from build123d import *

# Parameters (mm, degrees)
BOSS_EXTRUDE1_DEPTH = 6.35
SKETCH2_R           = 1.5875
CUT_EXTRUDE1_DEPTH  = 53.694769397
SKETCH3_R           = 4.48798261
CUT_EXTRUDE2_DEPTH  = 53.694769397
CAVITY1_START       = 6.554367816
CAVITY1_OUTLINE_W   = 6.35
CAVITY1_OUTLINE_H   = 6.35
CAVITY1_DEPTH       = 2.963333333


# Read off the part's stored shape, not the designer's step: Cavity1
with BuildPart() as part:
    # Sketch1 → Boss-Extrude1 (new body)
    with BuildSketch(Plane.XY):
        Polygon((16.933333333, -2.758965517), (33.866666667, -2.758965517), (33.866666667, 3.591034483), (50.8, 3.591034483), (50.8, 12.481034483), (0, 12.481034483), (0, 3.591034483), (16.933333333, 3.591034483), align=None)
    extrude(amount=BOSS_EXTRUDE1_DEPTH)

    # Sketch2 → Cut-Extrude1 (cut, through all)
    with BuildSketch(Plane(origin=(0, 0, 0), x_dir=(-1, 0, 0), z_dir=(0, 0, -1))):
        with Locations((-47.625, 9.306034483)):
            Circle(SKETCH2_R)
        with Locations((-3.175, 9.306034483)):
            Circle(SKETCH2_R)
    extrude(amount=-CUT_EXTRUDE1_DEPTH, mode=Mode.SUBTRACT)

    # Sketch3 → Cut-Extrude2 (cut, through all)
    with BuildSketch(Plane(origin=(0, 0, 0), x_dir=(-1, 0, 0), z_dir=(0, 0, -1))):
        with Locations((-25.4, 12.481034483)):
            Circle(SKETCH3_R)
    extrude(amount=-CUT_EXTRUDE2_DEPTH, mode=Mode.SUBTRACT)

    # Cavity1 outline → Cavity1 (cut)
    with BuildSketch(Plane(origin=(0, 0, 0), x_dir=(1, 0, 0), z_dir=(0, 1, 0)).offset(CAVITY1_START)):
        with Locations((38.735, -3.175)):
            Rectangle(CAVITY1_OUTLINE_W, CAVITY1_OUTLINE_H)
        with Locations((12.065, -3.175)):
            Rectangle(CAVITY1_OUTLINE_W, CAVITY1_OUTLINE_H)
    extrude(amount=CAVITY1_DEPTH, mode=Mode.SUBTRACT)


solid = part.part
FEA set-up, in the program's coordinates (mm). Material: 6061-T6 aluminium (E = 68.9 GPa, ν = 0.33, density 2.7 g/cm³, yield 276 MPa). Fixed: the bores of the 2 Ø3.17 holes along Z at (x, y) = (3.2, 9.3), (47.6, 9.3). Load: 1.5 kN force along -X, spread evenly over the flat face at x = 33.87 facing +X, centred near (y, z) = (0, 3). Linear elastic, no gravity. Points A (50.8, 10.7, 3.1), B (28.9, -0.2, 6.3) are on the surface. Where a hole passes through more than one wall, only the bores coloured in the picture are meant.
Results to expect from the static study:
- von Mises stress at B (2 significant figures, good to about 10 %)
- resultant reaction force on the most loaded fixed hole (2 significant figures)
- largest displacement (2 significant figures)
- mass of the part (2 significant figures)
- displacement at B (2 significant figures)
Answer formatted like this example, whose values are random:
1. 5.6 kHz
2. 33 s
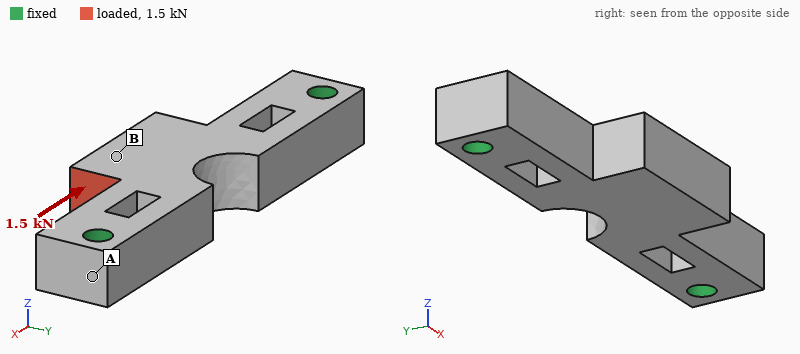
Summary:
1. 28 MPa
2. 810 N
3. 24 µm
4. 8.1 g
5. 15 µm
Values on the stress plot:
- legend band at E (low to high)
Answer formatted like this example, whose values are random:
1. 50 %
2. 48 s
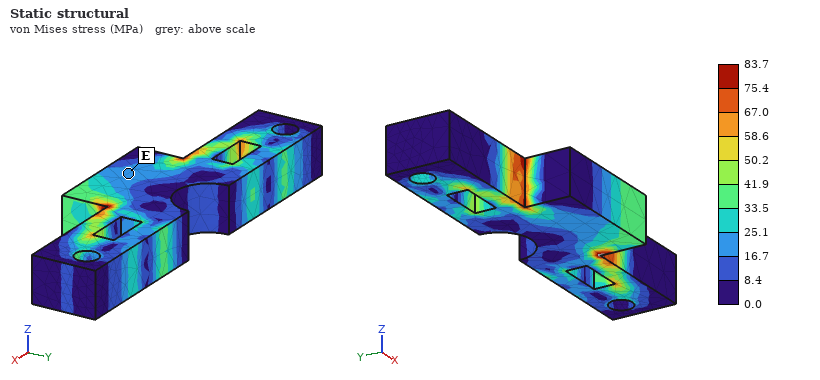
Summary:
1. 16.7 to 25.1 MPa
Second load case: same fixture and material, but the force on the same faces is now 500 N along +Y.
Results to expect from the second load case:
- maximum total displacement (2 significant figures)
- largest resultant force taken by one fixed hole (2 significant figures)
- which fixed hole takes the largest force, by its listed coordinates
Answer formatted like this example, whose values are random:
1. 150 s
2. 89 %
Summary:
1. 26 µm
2. 420 N
3. (47.6, 9.3)
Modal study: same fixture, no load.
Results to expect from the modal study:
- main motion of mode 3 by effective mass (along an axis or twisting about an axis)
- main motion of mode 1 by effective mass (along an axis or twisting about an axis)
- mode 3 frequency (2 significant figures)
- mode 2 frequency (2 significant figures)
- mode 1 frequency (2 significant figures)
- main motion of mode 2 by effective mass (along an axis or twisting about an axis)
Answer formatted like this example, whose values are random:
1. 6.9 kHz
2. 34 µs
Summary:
1. along Z
2. along Z
3. 20 kHz
4. 12 kHz
5. 9600 Hz
6. along Y
